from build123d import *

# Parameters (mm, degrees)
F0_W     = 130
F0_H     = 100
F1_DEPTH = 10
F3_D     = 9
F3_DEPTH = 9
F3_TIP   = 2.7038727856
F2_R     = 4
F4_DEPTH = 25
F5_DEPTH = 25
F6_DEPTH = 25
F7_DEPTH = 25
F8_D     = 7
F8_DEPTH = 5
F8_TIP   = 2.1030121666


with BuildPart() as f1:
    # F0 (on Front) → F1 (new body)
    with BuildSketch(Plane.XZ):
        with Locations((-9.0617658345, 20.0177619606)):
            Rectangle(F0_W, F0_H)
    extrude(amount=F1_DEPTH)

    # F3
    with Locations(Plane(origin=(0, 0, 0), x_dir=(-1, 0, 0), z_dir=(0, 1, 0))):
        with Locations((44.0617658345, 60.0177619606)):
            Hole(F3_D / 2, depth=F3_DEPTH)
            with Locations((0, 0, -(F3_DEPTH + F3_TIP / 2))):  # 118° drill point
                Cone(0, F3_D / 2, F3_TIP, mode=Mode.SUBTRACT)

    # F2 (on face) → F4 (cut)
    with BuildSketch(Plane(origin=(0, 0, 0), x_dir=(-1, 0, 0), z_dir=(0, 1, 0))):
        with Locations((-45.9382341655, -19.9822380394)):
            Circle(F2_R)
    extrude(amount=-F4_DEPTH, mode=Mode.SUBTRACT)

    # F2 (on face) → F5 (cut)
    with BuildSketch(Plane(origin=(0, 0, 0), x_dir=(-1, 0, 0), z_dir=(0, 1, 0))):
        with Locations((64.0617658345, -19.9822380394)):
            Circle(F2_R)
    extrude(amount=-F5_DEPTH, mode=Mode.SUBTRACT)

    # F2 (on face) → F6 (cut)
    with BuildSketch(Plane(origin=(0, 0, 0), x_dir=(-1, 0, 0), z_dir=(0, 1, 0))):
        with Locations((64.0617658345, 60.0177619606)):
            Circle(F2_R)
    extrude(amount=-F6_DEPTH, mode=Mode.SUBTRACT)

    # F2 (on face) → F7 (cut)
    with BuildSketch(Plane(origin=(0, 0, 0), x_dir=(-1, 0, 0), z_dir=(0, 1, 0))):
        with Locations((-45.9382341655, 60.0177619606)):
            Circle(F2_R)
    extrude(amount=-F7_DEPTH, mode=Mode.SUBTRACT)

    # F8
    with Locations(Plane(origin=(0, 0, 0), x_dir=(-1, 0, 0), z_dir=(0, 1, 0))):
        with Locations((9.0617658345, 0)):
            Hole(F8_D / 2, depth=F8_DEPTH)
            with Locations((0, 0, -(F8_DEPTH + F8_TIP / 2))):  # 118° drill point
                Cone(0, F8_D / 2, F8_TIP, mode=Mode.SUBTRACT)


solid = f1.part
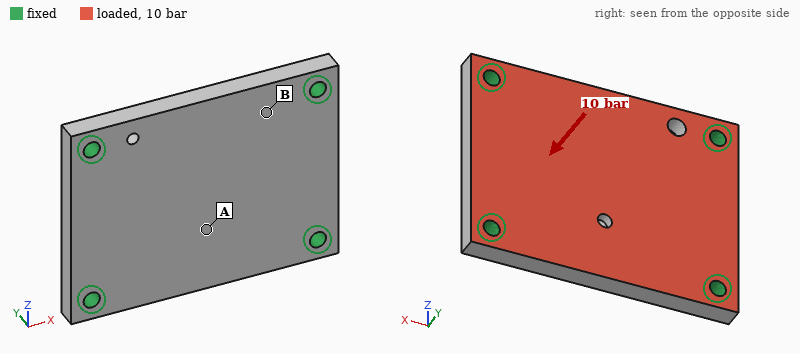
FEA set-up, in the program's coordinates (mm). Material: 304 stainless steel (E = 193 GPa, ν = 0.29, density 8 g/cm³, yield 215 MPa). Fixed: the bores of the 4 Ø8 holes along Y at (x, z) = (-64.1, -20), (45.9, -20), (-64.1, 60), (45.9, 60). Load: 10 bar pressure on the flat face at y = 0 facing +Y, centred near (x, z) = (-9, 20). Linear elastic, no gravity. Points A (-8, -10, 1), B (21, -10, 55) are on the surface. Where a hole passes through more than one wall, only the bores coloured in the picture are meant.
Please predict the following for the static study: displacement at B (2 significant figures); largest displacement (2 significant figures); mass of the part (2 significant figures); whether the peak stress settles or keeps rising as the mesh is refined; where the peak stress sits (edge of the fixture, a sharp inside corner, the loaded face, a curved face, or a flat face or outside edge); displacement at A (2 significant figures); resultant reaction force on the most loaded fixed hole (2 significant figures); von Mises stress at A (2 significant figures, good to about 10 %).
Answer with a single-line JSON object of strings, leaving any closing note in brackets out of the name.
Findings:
{"displacement at B": "19 µm", "largest displacement": "40 µm", "mass of the part": "1.0 kg", "whether the peak stress settles or keeps rising as the mesh is refined": "keeps rising", "where the peak stress sits": "edge of the fixture", "displacement at A": "38 µm", "resultant reaction force on the most loaded fixed hole": "3.2 kN", "von Mises stress at A": "33 MPa"}
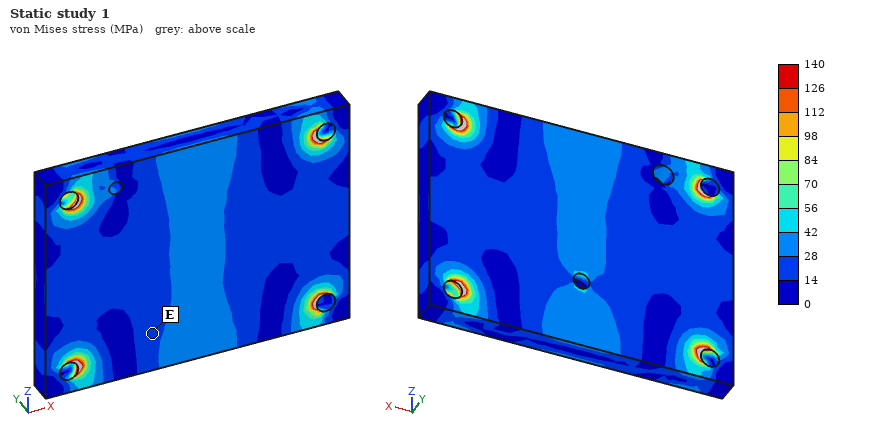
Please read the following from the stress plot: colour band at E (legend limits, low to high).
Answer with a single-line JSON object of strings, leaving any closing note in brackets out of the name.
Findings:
{"colour band at E": "14 to 28 MPa"}
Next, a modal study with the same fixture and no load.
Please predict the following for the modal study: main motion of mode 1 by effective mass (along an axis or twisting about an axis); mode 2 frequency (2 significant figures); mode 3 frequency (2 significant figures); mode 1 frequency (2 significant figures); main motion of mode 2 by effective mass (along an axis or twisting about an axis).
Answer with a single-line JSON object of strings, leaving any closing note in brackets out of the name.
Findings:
{"main motion of mode 1 by effective mass": "along Y", "mode 2 frequency": "4900 Hz", "mode 3 frequency": "7000 Hz", "mode 1 frequency": "3300 Hz", "main motion of mode 2 by effective mass": "twisting about X"}
